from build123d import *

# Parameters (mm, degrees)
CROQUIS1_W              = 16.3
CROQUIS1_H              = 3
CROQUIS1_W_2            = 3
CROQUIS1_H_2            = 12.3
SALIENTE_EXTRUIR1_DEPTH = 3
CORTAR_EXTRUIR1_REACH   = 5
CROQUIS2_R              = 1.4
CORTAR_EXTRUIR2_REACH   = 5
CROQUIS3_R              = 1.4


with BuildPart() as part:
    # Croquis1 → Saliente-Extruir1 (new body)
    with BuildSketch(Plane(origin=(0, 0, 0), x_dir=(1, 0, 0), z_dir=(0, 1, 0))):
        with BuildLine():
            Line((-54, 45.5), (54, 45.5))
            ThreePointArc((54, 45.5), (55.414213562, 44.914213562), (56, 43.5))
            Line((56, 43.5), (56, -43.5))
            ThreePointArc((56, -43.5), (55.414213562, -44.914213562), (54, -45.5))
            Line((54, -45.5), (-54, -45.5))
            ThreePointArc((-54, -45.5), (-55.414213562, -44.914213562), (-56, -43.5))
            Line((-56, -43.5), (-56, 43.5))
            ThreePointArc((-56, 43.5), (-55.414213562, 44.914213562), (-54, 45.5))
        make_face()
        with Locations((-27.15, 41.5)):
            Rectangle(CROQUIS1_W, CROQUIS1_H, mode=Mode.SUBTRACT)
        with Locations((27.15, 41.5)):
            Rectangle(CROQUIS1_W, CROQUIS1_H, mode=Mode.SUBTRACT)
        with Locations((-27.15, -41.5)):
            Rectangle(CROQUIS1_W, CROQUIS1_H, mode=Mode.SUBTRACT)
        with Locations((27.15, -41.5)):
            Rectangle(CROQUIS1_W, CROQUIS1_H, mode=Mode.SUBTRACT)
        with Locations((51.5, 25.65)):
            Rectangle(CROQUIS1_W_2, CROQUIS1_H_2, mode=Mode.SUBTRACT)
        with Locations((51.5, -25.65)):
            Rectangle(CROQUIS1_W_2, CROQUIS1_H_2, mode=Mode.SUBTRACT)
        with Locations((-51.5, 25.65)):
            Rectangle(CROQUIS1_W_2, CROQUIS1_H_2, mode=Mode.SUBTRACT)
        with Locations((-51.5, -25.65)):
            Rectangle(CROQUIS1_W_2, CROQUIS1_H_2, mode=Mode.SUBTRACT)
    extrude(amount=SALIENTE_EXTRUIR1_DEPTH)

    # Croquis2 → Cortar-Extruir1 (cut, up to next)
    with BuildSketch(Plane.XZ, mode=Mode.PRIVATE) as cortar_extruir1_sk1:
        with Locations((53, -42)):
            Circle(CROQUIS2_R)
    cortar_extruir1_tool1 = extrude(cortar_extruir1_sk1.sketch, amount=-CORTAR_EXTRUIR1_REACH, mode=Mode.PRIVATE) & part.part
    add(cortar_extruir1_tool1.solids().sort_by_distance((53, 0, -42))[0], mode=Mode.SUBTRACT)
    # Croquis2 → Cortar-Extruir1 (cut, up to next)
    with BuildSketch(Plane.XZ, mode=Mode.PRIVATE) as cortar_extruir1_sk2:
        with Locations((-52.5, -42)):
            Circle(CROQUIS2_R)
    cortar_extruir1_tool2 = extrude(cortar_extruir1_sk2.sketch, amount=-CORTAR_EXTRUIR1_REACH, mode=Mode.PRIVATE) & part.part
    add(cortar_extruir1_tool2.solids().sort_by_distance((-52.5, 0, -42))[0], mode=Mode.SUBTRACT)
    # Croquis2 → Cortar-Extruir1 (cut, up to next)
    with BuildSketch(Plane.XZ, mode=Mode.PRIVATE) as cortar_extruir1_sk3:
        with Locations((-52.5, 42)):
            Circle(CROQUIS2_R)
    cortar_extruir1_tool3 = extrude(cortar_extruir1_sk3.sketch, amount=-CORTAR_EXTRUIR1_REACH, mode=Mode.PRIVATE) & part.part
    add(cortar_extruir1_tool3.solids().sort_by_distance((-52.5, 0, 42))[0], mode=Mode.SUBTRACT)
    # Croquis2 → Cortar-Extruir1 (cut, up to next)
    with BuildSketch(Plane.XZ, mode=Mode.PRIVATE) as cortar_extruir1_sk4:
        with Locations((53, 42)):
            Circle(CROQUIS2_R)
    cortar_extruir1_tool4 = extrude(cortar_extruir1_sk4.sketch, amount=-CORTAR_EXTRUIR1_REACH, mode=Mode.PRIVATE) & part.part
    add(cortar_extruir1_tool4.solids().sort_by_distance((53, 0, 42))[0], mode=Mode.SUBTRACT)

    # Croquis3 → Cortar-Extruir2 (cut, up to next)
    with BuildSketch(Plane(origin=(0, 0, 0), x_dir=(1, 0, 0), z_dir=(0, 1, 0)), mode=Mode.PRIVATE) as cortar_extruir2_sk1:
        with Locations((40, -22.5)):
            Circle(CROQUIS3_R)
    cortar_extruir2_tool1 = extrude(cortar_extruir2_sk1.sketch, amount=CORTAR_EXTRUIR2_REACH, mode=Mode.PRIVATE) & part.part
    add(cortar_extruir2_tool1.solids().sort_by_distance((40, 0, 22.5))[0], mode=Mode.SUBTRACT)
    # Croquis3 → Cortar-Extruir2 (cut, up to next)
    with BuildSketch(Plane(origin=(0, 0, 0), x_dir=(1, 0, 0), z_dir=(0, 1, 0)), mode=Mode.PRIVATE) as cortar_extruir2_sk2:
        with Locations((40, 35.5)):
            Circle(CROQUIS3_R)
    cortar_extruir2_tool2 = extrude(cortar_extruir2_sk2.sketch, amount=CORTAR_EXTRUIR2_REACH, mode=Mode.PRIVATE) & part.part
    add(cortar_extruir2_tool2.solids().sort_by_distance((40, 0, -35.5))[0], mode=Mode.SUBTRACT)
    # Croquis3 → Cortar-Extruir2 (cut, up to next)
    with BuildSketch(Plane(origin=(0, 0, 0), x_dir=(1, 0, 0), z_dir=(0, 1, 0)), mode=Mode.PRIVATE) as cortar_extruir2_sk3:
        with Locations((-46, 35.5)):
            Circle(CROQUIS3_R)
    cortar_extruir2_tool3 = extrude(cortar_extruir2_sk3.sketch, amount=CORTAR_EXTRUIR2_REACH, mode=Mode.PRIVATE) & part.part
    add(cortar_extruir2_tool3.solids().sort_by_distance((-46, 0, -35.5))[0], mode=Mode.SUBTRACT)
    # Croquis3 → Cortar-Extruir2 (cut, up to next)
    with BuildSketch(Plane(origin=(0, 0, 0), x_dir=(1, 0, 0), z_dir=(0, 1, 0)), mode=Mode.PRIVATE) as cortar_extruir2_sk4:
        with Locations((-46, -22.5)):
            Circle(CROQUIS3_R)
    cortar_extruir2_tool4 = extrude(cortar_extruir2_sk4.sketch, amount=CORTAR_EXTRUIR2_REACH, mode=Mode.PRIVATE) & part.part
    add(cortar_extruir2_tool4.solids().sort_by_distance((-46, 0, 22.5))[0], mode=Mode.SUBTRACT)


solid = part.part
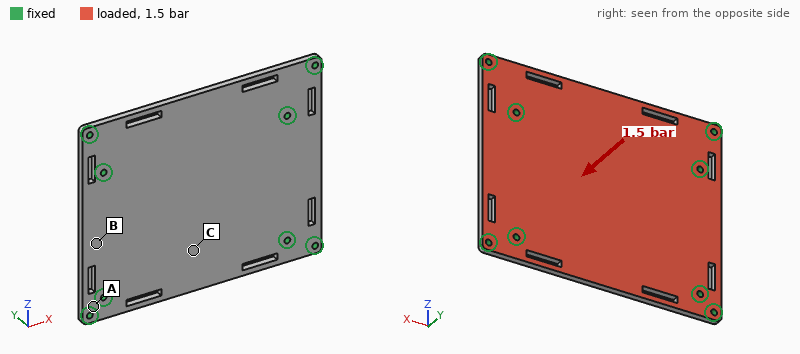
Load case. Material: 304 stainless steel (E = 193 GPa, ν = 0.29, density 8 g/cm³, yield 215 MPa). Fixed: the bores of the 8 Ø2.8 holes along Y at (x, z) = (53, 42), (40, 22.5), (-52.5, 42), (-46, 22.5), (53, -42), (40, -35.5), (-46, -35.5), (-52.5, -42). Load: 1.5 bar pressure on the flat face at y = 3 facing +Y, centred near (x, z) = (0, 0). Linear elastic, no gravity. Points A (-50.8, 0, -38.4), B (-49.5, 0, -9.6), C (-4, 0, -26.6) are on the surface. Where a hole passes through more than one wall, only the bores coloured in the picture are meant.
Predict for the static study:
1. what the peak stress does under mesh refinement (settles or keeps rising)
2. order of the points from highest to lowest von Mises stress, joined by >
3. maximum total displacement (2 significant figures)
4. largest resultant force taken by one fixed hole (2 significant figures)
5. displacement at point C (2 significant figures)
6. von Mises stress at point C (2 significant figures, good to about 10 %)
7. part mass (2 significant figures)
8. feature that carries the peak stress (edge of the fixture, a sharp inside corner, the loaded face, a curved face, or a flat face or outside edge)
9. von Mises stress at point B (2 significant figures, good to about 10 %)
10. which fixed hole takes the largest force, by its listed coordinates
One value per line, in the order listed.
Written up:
keeps rising
C > B > A
77 µm
460 N
71 µm
33 MPa
240 g
edge of the fixture
19 MPa
(40, 22.5)
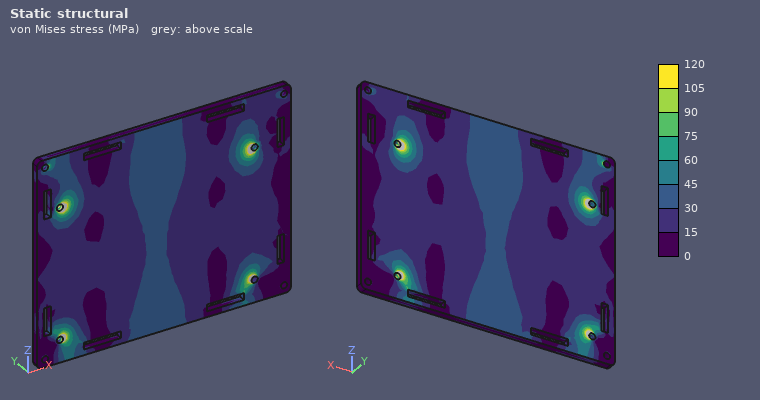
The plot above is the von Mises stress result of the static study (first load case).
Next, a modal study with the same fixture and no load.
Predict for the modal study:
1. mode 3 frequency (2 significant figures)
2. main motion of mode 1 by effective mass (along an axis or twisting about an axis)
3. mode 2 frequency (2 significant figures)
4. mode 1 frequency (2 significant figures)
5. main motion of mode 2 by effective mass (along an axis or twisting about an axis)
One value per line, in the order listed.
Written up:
3100 Hz
along Y
2100 Hz
1700 Hz
twisting about X
